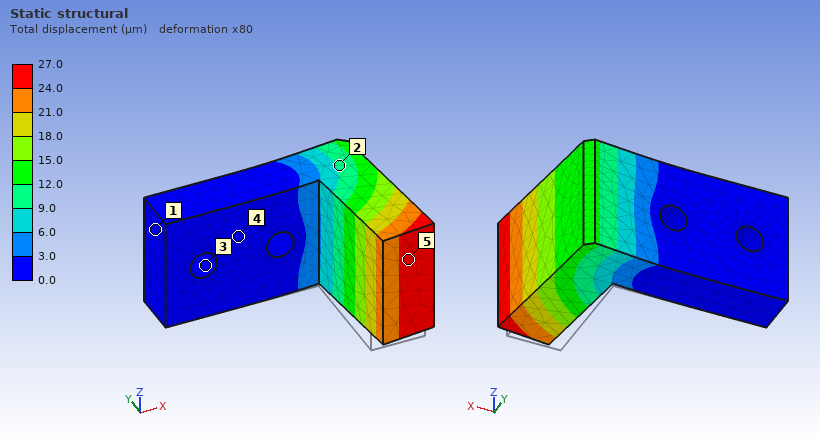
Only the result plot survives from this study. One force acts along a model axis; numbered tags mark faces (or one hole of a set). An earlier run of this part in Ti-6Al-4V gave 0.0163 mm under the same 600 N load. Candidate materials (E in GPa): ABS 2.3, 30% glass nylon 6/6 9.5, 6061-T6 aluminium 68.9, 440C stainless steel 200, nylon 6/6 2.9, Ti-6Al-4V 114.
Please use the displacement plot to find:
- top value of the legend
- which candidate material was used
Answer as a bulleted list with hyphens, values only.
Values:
- 27.0 µm
- 6061-T6 aluminium
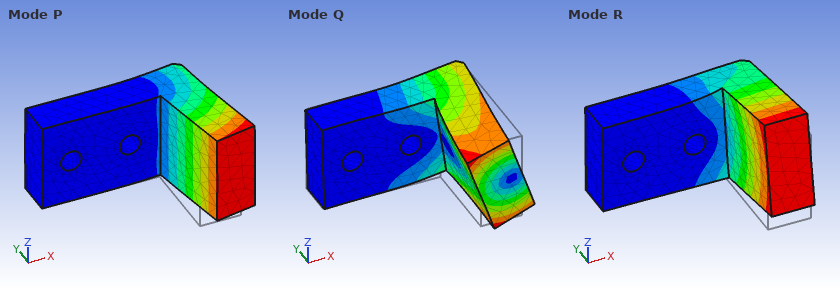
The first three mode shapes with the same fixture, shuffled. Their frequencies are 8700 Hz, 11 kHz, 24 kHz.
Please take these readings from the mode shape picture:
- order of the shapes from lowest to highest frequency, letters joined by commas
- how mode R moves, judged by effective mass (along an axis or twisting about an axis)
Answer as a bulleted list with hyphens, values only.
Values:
- P, R, Q
- along Z
